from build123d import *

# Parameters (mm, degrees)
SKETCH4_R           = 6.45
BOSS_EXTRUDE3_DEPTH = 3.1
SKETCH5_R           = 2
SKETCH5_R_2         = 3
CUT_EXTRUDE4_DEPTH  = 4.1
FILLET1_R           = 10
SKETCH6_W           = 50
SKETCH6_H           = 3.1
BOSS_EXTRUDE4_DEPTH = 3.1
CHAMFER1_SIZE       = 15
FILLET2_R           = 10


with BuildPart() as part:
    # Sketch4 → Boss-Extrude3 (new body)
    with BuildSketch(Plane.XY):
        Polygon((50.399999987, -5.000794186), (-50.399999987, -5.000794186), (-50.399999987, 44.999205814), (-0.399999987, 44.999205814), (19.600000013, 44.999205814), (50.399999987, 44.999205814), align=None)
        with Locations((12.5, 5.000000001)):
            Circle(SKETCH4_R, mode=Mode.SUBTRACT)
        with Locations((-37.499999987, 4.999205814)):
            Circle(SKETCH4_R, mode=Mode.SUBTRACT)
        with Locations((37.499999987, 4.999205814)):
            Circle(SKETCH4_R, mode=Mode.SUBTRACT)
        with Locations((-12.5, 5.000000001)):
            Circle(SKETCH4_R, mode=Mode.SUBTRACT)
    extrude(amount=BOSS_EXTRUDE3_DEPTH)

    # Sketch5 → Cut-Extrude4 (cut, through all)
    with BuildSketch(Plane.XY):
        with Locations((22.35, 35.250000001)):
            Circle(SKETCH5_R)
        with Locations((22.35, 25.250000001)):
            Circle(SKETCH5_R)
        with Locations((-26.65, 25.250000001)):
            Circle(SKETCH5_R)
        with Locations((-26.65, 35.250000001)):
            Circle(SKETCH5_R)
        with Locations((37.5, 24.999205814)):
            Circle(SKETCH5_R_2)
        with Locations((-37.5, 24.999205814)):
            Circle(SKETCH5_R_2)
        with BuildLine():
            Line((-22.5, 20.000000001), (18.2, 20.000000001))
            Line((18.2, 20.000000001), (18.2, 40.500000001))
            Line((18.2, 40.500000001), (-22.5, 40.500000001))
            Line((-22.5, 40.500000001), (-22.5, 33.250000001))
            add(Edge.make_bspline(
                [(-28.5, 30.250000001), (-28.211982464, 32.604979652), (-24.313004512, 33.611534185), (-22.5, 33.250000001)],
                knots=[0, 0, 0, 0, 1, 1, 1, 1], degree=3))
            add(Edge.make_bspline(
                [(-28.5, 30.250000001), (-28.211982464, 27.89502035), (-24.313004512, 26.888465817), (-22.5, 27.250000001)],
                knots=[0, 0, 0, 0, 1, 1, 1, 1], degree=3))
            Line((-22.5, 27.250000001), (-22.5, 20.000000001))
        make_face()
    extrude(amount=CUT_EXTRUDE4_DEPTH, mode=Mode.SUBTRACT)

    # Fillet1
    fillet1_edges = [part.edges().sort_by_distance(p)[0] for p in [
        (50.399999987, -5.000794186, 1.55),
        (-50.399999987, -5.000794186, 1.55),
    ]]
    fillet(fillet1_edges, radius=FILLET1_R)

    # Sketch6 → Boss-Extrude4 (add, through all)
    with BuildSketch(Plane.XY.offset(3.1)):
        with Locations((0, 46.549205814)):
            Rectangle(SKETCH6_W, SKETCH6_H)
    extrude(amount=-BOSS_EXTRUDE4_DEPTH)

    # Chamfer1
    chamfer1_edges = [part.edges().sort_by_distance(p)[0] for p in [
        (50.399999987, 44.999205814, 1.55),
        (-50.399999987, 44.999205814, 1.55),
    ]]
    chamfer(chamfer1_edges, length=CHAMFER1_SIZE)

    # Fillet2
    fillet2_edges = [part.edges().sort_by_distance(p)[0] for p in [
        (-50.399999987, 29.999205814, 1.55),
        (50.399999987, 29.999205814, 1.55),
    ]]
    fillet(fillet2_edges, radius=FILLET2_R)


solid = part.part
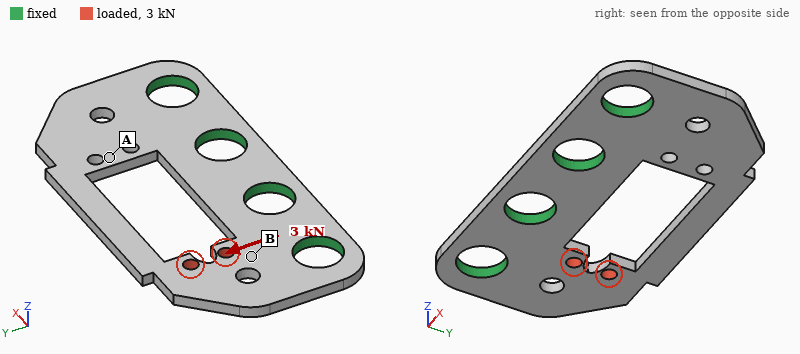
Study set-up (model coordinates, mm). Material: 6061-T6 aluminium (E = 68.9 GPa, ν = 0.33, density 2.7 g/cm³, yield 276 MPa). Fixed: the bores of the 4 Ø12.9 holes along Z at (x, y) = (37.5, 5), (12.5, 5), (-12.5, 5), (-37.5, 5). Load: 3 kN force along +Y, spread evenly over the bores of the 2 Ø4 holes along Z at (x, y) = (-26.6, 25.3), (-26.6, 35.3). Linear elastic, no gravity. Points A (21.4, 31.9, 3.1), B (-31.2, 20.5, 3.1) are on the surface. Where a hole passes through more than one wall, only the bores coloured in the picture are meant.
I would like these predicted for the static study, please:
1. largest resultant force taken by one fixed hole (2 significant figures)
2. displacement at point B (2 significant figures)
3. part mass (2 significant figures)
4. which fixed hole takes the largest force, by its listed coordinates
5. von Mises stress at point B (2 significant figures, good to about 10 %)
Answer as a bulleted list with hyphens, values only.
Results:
- 2.3 kN
- 9.4 µm
- 29 g
- (-37.5, 5)
- 73 MPa
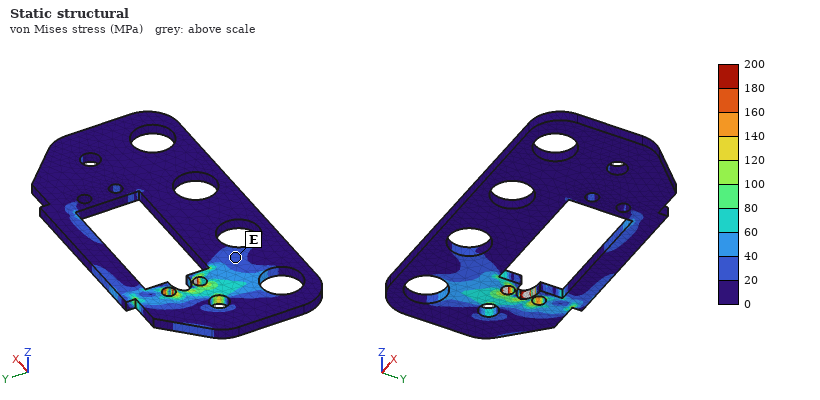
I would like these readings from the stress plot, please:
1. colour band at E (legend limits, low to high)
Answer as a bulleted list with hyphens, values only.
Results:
- 20 to 40 MPa
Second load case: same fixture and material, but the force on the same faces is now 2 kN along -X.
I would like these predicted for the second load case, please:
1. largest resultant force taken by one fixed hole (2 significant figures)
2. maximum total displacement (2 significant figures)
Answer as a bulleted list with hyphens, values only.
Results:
- 1.1 kN
- 39 µm
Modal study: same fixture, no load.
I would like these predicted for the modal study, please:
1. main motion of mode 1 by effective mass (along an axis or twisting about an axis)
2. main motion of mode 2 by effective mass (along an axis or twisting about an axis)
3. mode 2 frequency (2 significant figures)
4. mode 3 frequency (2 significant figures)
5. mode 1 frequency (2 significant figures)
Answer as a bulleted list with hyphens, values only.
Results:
- along Z
- twisting about Y
- 2700 Hz
- 4500 Hz
- 1600 Hz
